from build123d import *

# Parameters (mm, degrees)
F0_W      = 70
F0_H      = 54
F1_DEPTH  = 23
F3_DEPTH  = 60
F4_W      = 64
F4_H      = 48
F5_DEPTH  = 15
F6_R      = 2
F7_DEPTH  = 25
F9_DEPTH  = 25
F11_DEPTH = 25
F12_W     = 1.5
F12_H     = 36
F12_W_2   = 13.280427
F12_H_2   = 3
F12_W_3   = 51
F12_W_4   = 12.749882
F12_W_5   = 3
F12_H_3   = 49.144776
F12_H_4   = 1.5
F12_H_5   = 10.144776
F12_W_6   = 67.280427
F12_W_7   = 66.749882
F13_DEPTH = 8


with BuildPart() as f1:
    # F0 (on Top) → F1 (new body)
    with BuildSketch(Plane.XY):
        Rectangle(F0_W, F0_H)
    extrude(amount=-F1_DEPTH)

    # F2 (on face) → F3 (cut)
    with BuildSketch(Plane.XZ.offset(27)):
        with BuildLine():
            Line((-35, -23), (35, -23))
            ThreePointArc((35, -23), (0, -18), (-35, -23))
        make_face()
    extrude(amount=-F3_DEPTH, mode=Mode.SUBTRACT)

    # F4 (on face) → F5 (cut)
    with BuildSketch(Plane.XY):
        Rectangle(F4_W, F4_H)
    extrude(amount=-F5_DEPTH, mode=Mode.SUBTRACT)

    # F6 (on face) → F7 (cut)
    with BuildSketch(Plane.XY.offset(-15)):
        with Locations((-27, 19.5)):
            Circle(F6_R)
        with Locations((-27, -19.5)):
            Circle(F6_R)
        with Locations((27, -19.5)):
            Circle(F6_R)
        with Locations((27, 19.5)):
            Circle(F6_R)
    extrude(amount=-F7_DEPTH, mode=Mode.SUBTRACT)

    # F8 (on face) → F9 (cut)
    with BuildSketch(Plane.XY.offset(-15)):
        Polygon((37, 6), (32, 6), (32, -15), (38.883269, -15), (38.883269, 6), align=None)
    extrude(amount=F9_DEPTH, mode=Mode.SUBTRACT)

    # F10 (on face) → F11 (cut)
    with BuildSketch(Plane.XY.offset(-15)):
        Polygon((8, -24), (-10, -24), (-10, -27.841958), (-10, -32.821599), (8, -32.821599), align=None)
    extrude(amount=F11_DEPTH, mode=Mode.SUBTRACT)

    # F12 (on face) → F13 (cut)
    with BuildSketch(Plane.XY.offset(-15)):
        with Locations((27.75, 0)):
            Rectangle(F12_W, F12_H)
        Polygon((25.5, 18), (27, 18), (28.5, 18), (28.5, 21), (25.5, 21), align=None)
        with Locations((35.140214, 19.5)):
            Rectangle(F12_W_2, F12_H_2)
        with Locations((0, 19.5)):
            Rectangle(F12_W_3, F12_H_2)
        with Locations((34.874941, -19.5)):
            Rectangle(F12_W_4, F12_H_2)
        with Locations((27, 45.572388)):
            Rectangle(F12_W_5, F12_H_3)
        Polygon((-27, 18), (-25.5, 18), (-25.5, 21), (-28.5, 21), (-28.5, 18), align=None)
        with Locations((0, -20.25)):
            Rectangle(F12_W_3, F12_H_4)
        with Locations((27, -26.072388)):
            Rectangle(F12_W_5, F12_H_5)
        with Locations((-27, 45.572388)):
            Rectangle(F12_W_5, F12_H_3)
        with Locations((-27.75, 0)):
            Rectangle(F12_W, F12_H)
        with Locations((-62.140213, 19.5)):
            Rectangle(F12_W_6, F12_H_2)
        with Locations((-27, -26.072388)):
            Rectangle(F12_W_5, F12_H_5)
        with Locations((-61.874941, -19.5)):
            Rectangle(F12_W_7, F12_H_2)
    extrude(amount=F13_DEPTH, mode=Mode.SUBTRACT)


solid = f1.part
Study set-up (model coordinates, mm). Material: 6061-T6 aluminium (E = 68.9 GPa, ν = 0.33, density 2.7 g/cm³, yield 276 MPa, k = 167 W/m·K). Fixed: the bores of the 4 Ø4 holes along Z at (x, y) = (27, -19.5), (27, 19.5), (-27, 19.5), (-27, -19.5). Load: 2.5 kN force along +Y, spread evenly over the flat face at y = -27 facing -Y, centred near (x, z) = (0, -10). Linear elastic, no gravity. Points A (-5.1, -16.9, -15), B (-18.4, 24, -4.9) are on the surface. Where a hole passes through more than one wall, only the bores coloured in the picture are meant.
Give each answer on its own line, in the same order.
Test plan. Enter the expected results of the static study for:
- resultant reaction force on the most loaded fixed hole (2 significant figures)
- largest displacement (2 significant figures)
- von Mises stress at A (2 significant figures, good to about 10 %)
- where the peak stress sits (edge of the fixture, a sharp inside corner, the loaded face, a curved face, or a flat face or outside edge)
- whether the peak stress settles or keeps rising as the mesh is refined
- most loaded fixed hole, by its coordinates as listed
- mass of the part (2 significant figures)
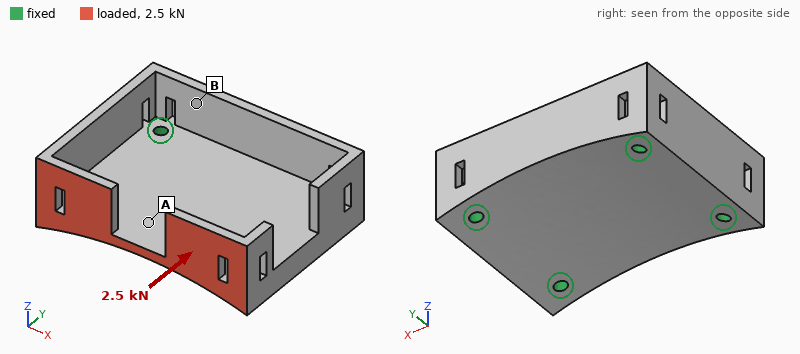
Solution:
970 N
0.16 mm
21 MPa
edge of the fixture
keeps rising
(27, -19.5)
69 g
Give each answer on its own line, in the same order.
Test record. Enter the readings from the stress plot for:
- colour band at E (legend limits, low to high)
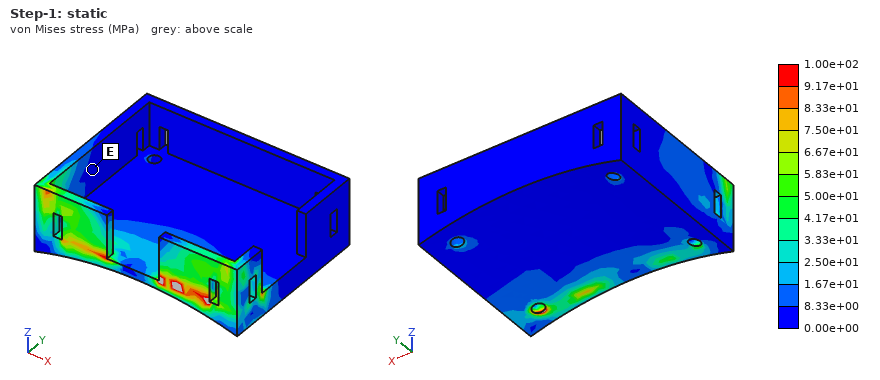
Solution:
0.00e+00 to 8.33e+00 MPa
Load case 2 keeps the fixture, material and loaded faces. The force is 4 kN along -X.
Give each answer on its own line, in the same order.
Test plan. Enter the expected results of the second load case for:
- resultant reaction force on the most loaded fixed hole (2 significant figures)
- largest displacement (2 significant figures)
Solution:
2.0 kN
64 µm
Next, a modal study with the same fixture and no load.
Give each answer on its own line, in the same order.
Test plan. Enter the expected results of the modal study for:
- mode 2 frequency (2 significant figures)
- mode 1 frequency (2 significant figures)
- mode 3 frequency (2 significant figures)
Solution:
8400 Hz
7600 Hz
9000 Hz
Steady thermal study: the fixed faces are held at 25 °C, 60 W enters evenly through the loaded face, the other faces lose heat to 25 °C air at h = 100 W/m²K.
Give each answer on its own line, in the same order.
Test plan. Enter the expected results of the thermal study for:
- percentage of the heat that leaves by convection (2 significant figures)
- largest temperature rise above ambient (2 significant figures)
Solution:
9.8 %
25 K
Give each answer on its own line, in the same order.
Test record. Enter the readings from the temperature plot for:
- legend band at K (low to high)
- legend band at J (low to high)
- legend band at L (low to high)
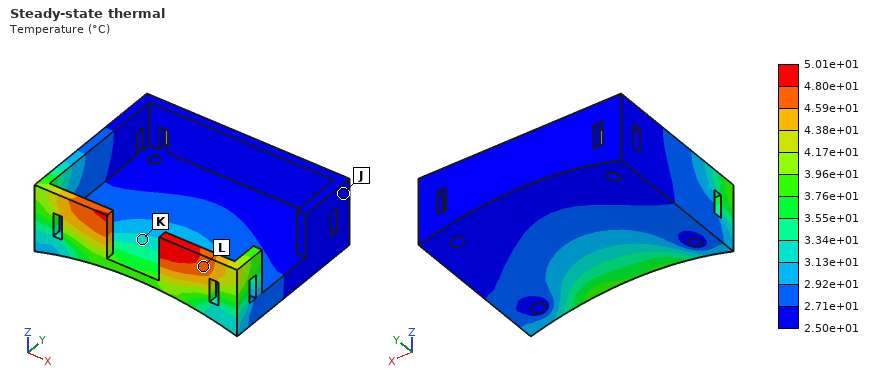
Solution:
3.13e+01 to 3.34e+01 °C
2.50e+01 to 2.71e+01 °C
4.59e+01 to 4.80e+01 °C
